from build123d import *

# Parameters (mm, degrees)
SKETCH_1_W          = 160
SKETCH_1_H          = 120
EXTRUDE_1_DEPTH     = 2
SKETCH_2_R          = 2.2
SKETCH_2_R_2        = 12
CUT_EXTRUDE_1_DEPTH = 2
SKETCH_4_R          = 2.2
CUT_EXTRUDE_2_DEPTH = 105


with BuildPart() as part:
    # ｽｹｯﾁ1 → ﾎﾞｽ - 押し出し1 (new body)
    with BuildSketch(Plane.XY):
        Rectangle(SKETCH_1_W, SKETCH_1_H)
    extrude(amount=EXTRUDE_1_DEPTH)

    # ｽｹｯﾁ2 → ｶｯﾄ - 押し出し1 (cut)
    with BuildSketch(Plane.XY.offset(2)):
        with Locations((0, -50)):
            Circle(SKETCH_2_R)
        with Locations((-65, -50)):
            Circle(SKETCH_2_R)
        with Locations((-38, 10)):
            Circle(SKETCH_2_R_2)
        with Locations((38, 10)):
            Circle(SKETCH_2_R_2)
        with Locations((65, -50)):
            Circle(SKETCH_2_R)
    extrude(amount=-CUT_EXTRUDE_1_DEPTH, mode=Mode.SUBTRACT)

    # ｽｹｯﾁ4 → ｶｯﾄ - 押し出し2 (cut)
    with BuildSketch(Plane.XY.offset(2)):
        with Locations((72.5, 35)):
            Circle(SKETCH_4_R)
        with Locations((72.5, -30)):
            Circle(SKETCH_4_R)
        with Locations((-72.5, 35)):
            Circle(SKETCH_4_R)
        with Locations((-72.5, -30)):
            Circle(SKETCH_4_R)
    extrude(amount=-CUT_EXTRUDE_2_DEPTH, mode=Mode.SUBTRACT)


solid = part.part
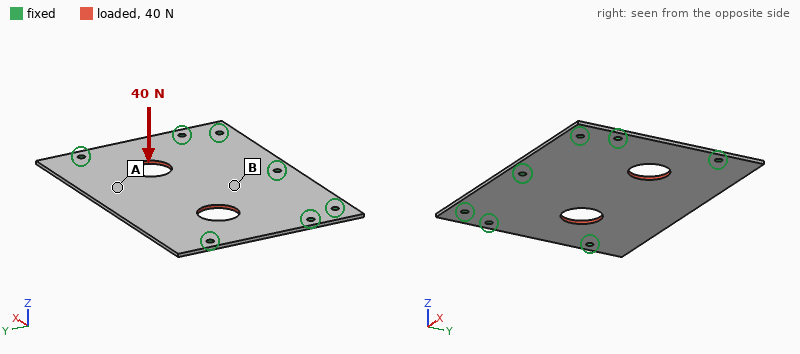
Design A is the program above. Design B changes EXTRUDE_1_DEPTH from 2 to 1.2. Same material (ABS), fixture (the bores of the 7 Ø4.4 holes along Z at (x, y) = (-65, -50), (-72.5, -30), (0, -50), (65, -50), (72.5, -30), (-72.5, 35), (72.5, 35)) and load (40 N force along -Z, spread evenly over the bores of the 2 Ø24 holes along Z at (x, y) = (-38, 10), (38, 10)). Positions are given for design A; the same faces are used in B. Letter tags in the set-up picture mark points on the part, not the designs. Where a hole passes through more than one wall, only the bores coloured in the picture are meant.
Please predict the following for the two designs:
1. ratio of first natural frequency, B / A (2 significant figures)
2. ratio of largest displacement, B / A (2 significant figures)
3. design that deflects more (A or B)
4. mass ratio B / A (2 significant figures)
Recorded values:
0.61
4.5
B
0.60
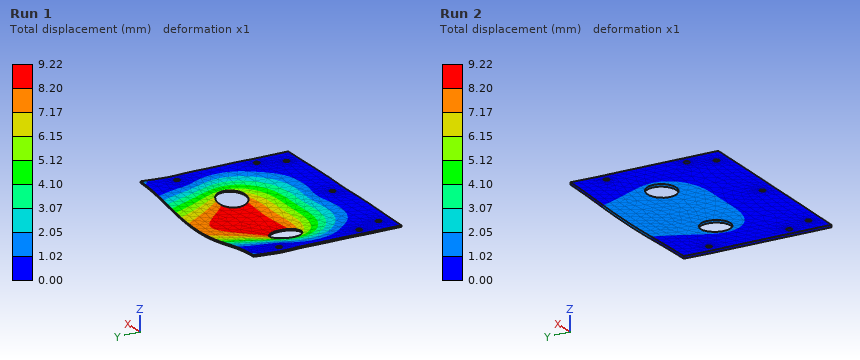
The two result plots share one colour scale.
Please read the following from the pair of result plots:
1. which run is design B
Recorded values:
Run 1
